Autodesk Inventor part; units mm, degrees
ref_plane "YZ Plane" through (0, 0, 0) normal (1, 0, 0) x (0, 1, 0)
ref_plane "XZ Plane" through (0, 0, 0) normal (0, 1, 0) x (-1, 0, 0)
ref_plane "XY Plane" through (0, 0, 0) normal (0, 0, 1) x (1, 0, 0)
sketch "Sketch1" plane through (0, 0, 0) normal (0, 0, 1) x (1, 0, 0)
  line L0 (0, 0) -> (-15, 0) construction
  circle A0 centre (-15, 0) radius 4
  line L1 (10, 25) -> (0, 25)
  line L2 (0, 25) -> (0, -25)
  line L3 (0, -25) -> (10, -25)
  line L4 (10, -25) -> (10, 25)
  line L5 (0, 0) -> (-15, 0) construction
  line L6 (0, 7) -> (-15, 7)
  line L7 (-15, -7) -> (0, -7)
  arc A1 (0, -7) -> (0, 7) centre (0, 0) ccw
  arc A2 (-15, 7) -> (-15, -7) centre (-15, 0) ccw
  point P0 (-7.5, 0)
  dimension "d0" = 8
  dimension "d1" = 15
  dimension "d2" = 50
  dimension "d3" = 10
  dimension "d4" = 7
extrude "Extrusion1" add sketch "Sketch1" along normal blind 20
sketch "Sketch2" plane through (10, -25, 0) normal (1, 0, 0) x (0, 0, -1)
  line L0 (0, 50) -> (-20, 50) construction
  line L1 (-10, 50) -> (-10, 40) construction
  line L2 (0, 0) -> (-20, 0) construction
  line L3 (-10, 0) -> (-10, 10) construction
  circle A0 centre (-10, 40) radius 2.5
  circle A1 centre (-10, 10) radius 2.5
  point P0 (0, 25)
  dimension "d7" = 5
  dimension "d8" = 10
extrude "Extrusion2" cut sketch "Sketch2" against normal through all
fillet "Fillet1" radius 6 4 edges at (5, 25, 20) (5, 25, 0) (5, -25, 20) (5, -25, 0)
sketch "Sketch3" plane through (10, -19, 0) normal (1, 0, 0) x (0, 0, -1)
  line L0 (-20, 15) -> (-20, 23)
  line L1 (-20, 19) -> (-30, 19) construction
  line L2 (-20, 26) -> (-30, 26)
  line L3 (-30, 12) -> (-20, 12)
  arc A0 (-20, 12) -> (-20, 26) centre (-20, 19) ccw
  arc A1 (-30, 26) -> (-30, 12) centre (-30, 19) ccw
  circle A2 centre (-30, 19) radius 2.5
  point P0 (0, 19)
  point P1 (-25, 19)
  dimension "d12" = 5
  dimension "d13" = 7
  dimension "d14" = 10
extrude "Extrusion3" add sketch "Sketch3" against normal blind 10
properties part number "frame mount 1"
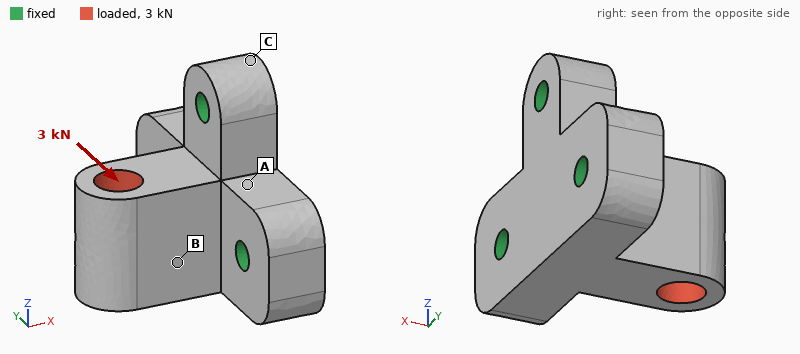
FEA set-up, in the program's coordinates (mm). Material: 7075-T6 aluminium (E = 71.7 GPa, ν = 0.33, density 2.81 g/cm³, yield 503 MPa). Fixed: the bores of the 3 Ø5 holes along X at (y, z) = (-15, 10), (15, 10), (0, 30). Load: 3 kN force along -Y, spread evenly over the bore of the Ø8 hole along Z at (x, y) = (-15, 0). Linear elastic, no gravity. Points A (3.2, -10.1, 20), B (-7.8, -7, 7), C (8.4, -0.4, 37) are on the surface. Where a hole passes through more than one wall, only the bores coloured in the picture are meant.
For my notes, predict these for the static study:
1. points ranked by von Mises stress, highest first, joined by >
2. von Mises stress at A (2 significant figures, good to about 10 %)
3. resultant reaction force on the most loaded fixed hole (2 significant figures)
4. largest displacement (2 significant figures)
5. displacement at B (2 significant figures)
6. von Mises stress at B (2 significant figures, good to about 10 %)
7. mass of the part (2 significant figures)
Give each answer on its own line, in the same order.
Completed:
B > A > C
20 MPa
2.7 kN
57 µm
21 µm
45 MPa
45 g
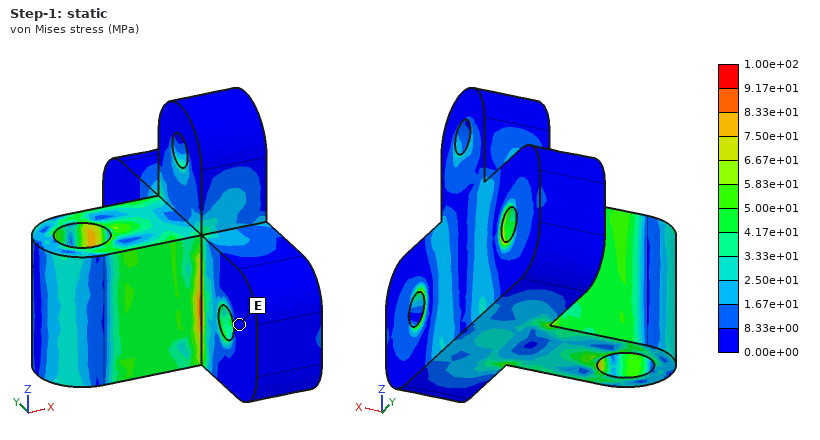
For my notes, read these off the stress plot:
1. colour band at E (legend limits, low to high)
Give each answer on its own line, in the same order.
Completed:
0.00e+00 to 8.33e+00 MPa
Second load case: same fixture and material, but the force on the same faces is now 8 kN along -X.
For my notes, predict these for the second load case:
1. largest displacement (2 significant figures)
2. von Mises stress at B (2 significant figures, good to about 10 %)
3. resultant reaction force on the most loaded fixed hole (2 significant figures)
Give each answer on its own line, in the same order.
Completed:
35 µm
44 MPa
3.5 kN
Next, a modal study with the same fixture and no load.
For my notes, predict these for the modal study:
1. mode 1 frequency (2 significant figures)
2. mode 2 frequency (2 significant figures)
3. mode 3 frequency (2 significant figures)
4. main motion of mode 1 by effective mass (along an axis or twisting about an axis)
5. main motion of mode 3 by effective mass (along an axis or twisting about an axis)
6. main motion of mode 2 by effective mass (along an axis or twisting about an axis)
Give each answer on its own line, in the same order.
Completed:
15 kHz
16 kHz
28 kHz
along Z
along X
along Y
